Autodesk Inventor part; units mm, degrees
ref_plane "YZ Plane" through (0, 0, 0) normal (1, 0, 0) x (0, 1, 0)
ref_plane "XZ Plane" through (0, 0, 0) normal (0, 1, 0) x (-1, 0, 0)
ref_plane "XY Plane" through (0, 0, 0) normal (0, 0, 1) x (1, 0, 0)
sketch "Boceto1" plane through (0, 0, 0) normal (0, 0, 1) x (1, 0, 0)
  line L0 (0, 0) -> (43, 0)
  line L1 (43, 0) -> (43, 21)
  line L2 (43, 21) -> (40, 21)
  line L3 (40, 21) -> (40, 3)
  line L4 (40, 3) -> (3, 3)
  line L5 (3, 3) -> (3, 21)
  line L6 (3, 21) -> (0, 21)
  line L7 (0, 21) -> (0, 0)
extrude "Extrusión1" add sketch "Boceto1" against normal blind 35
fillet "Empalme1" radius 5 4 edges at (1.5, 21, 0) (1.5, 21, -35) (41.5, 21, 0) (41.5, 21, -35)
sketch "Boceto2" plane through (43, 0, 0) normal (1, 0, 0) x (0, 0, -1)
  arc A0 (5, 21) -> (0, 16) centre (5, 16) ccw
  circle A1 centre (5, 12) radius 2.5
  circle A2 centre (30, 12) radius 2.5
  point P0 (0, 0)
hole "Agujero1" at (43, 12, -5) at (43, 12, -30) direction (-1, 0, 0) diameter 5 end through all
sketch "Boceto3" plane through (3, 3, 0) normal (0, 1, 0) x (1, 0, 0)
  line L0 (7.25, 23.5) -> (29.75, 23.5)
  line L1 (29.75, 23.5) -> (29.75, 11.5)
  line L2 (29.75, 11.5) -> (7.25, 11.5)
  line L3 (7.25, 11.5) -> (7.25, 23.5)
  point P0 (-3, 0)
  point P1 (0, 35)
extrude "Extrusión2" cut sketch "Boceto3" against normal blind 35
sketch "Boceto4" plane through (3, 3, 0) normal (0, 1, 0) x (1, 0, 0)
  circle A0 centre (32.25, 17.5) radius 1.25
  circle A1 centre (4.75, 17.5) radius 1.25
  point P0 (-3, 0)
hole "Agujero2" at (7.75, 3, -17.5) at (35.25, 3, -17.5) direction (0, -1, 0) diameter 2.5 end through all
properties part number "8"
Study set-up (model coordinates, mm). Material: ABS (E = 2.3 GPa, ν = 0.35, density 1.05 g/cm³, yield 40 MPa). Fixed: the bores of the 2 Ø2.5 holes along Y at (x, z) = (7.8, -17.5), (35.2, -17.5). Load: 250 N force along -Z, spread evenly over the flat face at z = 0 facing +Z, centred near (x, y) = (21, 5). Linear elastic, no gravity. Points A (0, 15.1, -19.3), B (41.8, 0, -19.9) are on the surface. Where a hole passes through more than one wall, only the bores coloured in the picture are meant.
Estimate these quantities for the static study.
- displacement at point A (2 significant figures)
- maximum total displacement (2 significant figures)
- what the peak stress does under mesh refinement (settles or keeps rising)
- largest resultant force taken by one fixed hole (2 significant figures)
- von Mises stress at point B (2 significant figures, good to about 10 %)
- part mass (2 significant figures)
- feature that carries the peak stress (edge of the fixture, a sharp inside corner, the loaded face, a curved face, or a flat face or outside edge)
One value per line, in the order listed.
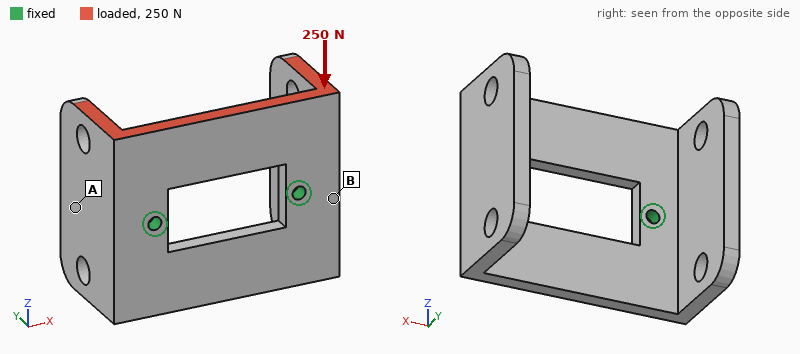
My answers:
0.25 mm
0.44 mm
keeps rising
130 N
3.8 MPa
7.5 g
edge of the fixture
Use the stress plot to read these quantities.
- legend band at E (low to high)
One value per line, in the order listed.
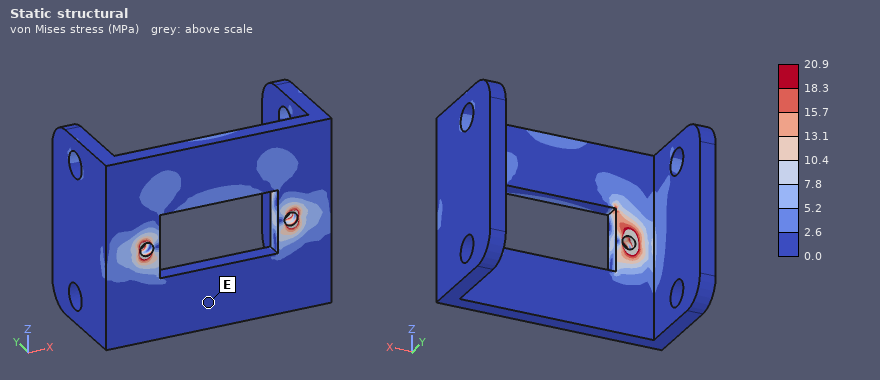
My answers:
0.0 to 2.6 MPa
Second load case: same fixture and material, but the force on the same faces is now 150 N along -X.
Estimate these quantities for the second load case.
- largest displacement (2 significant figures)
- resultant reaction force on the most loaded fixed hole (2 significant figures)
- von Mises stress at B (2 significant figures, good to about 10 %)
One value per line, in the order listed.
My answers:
0.55 mm
110 N
3.6 MPa
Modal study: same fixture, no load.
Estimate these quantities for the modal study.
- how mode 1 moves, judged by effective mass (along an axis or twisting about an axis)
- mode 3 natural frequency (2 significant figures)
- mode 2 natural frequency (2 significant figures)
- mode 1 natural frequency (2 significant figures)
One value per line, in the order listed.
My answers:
along Z
1200 Hz
1100 Hz
960 Hz
